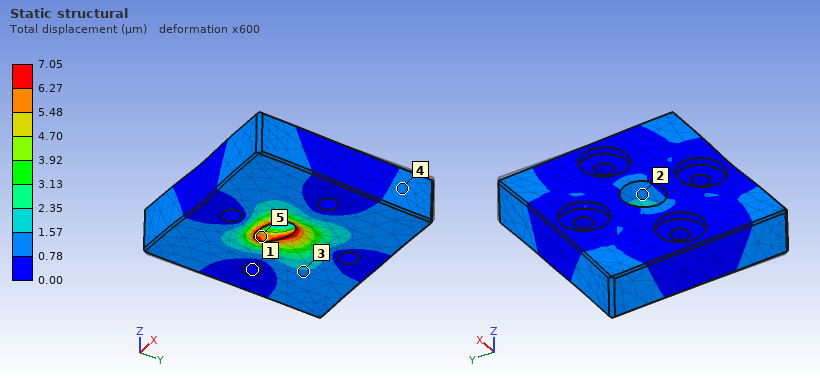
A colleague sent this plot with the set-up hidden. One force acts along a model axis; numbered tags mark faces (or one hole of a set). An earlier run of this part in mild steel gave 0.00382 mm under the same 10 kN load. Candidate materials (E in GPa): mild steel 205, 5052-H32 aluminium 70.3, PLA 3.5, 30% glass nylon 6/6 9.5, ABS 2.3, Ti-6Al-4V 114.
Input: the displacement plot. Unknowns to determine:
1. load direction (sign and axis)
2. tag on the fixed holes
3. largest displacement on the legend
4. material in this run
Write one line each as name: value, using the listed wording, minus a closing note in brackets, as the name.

load direction: -Y
tag on the fixed holes: 1
largest displacement on the legend: 7.05 µm
material in this run: Ti-6Al-4V
